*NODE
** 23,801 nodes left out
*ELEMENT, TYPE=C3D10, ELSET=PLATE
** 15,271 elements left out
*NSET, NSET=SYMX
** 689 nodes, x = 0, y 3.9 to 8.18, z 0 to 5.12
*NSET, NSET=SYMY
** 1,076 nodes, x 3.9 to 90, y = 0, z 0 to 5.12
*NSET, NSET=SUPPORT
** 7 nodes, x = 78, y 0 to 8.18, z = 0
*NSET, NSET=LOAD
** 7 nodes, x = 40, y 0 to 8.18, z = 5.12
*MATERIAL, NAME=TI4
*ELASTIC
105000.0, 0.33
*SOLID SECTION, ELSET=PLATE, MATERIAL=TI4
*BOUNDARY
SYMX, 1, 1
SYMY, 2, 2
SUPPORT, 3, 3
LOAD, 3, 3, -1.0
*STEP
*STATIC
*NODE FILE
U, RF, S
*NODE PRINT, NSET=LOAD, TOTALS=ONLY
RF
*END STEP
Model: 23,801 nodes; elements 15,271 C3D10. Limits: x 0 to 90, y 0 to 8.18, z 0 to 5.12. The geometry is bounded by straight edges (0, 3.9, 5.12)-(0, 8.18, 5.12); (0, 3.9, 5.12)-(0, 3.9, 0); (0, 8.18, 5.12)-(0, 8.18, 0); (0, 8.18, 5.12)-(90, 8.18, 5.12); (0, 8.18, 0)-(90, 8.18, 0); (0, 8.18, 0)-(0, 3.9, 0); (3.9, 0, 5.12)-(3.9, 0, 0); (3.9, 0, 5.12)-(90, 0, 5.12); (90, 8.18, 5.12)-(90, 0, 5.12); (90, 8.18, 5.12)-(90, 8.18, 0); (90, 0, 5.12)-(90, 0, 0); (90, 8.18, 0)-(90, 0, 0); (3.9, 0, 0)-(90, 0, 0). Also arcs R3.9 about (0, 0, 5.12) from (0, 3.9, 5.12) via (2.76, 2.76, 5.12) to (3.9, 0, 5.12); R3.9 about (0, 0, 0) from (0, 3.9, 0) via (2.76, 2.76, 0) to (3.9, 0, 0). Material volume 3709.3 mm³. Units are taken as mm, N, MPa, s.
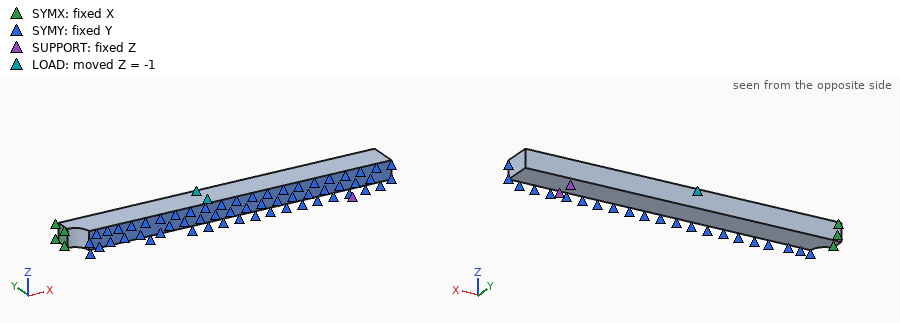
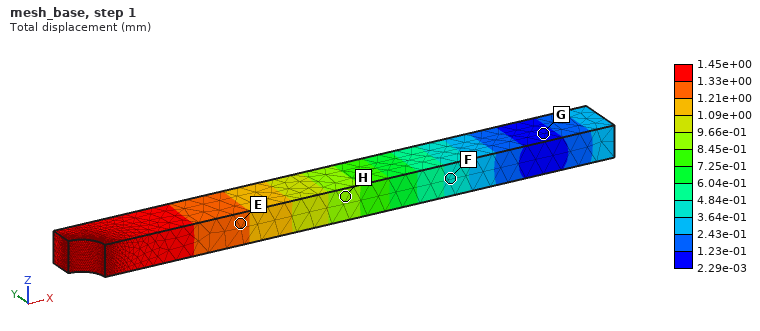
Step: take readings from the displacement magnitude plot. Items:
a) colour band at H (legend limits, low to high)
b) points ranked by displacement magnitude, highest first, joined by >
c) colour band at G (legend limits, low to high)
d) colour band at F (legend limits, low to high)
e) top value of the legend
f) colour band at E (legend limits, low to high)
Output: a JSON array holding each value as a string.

["8.45e-01 to 9.66e-01 mm", "E > H > F > G", "2.29e-03 to 1.23e-01 mm", "3.64e-01 to 4.84e-01 mm", "1.45e+00 mm", "1.21e+00 to 1.33e+00 mm"]
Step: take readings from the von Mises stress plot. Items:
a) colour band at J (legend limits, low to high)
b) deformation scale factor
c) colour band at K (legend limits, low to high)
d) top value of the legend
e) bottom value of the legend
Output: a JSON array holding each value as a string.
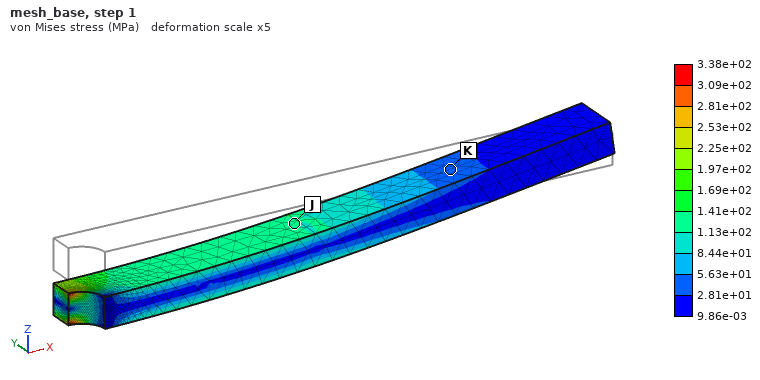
["1.13e+02 to 1.41e+02 MPa", "5", "2.81e+01 to 5.63e+01 MPa", "3.38e+02 MPa", "9.86e-03 MPa"]
